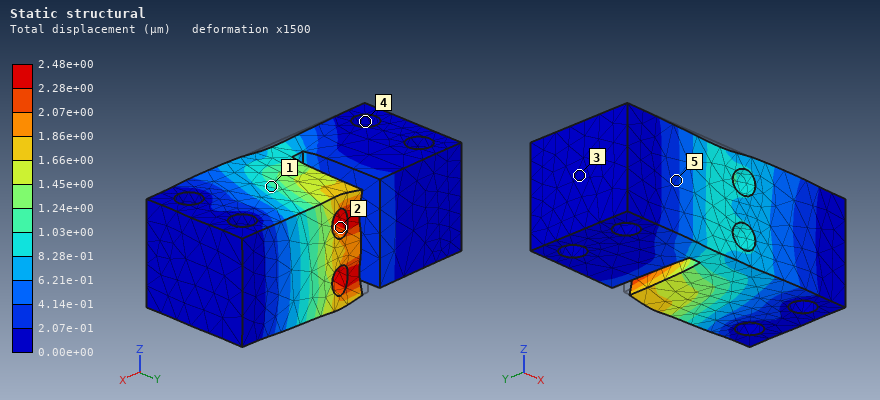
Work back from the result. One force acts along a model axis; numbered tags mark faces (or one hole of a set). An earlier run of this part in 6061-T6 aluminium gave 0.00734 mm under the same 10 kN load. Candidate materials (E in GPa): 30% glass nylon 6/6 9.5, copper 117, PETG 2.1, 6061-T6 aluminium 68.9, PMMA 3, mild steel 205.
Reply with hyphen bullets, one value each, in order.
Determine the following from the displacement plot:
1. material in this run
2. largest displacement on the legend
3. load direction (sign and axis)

- mild steel
- 2.48e+00 µm
- +X
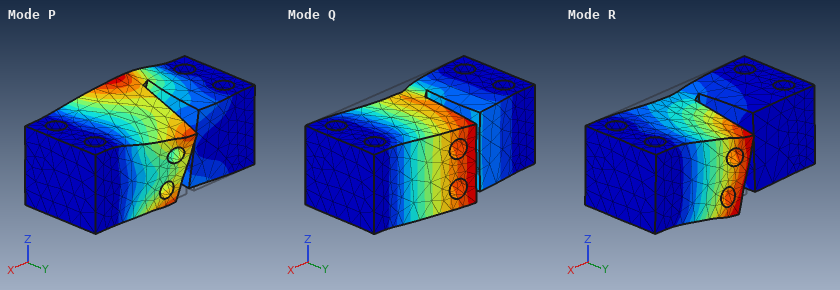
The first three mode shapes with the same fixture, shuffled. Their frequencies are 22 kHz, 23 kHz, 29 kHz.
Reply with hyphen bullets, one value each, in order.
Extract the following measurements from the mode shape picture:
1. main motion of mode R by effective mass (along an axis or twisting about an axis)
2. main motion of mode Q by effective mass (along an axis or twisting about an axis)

- along Z
- along Y
